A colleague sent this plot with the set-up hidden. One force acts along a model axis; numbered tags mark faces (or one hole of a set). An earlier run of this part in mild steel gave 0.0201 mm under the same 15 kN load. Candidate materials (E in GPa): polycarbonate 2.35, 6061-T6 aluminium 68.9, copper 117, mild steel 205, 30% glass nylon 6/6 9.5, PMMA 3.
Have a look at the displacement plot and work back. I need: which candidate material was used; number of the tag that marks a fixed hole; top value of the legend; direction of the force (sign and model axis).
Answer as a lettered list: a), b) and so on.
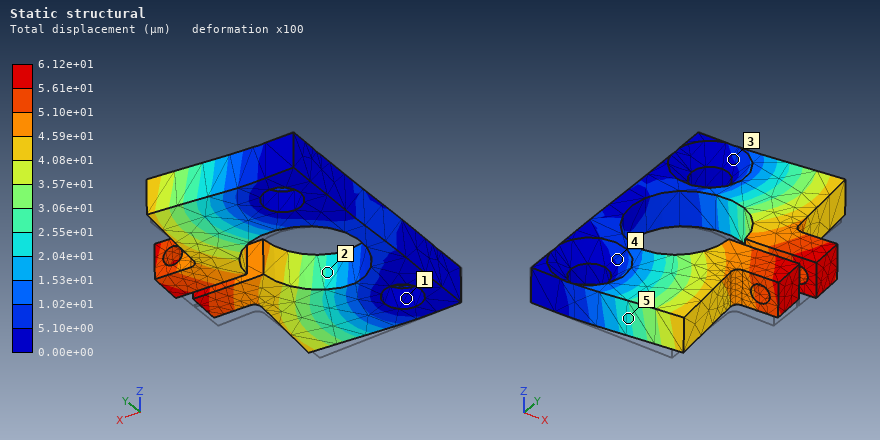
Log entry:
a) 6061-T6 aluminium
b) 1
c) 6.12e+01 µm
d) +Y
